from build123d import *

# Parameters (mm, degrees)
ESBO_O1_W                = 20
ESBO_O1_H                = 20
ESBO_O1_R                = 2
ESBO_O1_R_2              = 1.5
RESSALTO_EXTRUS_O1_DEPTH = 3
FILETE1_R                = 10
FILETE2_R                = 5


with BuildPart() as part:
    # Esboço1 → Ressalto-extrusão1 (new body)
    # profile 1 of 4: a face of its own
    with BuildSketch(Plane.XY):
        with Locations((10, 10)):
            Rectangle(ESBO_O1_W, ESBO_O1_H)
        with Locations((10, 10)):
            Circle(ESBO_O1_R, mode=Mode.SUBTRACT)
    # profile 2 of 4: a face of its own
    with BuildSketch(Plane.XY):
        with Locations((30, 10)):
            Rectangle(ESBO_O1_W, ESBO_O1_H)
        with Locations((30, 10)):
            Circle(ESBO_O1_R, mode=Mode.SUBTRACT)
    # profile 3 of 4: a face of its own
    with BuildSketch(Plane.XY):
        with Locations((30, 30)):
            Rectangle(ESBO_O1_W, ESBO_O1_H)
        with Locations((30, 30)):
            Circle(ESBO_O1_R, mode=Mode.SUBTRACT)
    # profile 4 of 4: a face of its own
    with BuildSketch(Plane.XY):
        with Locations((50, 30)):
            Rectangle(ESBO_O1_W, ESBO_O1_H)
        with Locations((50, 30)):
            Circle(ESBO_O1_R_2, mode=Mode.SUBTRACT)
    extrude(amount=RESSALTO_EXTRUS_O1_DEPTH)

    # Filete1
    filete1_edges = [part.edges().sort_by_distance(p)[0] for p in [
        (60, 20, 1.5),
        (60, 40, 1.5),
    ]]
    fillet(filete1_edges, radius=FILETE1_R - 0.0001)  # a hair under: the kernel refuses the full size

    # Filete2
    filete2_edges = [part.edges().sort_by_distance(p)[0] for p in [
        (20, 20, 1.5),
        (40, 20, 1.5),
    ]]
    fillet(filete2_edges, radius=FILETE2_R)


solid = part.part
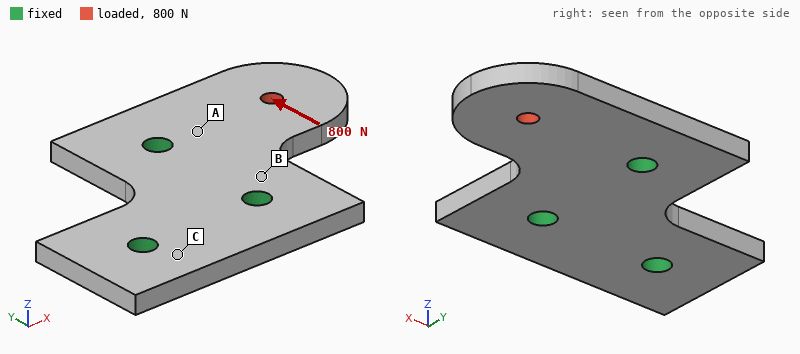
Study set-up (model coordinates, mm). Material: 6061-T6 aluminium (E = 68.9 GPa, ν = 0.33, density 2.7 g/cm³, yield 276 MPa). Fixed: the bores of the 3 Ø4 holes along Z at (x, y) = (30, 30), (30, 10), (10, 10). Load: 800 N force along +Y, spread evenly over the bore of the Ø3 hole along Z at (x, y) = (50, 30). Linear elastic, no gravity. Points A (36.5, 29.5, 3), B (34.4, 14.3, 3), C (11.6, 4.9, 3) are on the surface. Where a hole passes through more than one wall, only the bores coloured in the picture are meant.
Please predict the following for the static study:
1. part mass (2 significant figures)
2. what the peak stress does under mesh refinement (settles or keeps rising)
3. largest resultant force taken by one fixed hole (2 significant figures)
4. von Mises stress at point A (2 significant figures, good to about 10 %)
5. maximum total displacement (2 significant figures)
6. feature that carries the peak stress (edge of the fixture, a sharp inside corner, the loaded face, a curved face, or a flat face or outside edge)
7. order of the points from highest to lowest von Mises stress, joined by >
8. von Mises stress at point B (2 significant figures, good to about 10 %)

12 g
keeps rising
780 N
21 MPa
32 µm
edge of the fixture
B > A > C
36 MPa
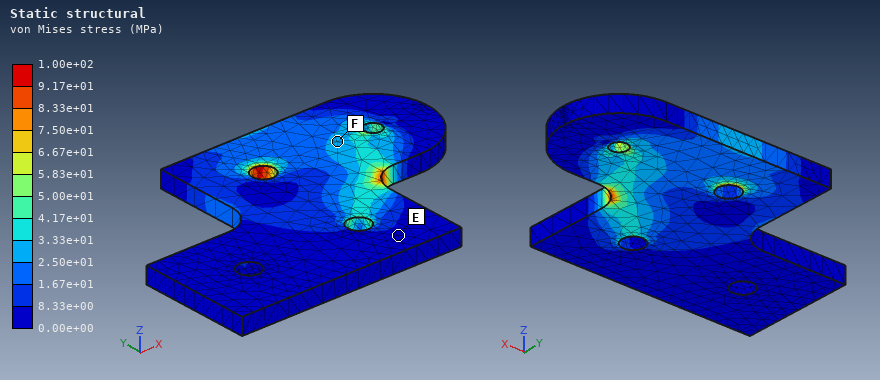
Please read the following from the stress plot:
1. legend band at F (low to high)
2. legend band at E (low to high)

2.50e+01 to 3.33e+01 MPa
0.00e+00 to 8.33e+00 MPa
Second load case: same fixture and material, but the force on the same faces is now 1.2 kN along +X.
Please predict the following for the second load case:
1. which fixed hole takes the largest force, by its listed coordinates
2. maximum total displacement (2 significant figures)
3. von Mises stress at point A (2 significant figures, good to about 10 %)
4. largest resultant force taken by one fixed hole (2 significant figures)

(30, 30)
11 µm
32 MPa
1.1 kN
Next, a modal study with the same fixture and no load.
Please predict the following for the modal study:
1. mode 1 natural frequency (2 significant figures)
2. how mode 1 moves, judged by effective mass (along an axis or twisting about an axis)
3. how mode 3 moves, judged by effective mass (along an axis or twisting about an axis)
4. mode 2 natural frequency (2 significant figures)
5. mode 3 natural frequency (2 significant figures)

3500 Hz
along Z
along Y
10 kHz
17 kHz
